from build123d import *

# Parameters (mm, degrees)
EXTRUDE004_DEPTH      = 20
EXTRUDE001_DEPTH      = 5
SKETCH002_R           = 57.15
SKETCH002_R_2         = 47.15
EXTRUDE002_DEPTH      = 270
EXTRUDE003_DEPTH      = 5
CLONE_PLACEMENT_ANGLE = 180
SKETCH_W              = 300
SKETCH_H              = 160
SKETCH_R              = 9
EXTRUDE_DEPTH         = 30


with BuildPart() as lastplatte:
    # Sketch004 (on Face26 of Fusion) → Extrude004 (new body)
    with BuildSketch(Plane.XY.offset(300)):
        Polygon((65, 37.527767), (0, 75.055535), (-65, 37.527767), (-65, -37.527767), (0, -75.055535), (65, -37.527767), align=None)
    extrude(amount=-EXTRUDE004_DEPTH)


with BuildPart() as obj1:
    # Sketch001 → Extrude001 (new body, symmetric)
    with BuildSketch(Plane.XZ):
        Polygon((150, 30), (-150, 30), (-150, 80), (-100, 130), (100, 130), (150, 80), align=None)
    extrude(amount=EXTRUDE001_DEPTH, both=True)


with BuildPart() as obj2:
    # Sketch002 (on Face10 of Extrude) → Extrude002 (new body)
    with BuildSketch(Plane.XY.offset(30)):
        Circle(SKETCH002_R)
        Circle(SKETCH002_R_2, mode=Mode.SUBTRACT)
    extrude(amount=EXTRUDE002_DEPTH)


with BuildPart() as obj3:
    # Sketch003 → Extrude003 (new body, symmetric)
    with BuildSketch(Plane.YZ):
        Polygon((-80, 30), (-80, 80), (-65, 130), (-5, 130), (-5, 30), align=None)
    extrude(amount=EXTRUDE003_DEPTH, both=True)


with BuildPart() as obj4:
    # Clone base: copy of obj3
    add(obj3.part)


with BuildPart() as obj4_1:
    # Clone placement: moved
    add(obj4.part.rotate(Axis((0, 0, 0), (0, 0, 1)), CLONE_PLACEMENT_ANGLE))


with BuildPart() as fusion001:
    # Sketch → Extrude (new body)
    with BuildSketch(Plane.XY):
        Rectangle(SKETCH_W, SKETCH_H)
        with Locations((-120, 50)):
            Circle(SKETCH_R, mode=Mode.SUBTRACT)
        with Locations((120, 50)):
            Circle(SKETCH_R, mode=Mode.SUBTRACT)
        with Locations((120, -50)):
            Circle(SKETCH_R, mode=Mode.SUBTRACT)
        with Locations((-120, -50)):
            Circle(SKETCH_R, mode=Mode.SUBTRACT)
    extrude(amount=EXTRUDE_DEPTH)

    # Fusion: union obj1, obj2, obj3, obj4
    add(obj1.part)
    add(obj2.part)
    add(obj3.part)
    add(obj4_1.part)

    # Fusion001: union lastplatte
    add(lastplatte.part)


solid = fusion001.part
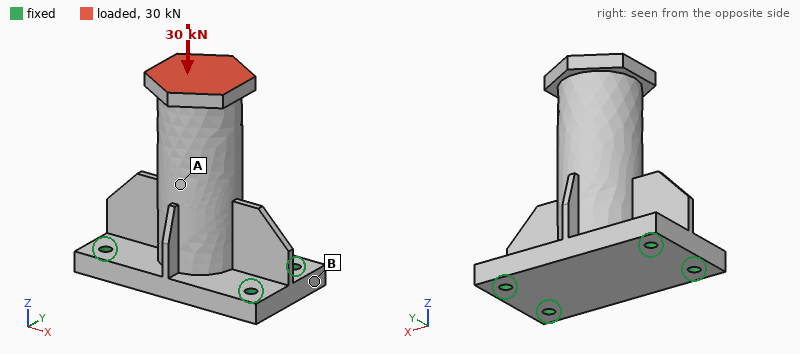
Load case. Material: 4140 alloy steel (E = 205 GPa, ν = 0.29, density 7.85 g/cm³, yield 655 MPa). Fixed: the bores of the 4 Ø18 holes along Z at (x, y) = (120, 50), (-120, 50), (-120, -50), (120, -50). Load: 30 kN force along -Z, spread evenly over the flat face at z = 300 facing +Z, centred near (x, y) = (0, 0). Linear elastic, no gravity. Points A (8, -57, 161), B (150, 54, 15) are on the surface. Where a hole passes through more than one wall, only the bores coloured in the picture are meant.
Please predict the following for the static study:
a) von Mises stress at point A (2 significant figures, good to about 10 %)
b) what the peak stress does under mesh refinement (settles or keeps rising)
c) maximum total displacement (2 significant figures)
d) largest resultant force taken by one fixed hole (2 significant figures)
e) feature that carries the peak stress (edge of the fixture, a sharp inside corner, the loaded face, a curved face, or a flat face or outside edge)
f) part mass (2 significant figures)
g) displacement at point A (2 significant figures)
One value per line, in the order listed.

7.3 MPa
keeps rising
24 µm
8.0 kN
edge of the fixture
23 kg
15 µm
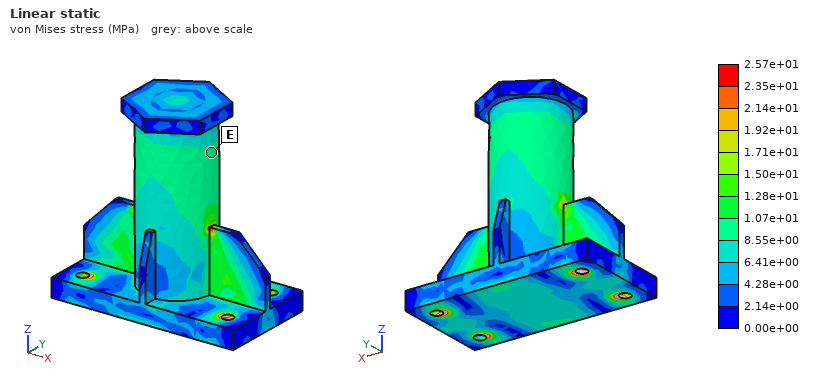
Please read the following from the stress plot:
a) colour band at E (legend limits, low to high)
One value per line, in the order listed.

8.55e+00 to 1.07e+01 MPa
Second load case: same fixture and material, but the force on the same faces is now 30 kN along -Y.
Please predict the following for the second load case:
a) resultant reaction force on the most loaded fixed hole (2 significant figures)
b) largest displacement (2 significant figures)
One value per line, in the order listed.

40 kN
0.74 mm
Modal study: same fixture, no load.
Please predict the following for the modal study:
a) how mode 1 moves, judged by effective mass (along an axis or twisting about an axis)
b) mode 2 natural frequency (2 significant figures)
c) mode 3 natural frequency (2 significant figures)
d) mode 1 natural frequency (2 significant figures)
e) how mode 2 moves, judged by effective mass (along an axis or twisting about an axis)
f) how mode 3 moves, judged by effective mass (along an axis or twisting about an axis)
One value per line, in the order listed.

along Y
980 Hz
1900 Hz
500 Hz
along X
along Z
